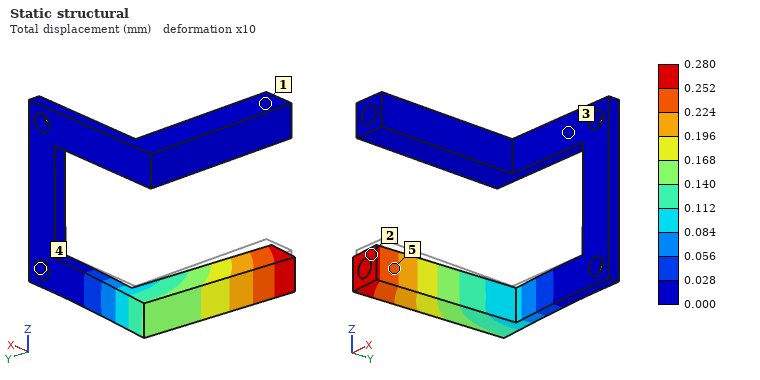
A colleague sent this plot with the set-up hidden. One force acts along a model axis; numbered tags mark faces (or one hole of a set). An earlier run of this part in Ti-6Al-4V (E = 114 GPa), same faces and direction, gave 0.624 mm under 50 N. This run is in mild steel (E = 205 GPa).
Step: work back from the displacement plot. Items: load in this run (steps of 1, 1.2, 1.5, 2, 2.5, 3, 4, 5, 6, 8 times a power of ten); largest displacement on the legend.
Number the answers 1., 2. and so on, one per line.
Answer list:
1. 40 N
2. 0.280 mm
